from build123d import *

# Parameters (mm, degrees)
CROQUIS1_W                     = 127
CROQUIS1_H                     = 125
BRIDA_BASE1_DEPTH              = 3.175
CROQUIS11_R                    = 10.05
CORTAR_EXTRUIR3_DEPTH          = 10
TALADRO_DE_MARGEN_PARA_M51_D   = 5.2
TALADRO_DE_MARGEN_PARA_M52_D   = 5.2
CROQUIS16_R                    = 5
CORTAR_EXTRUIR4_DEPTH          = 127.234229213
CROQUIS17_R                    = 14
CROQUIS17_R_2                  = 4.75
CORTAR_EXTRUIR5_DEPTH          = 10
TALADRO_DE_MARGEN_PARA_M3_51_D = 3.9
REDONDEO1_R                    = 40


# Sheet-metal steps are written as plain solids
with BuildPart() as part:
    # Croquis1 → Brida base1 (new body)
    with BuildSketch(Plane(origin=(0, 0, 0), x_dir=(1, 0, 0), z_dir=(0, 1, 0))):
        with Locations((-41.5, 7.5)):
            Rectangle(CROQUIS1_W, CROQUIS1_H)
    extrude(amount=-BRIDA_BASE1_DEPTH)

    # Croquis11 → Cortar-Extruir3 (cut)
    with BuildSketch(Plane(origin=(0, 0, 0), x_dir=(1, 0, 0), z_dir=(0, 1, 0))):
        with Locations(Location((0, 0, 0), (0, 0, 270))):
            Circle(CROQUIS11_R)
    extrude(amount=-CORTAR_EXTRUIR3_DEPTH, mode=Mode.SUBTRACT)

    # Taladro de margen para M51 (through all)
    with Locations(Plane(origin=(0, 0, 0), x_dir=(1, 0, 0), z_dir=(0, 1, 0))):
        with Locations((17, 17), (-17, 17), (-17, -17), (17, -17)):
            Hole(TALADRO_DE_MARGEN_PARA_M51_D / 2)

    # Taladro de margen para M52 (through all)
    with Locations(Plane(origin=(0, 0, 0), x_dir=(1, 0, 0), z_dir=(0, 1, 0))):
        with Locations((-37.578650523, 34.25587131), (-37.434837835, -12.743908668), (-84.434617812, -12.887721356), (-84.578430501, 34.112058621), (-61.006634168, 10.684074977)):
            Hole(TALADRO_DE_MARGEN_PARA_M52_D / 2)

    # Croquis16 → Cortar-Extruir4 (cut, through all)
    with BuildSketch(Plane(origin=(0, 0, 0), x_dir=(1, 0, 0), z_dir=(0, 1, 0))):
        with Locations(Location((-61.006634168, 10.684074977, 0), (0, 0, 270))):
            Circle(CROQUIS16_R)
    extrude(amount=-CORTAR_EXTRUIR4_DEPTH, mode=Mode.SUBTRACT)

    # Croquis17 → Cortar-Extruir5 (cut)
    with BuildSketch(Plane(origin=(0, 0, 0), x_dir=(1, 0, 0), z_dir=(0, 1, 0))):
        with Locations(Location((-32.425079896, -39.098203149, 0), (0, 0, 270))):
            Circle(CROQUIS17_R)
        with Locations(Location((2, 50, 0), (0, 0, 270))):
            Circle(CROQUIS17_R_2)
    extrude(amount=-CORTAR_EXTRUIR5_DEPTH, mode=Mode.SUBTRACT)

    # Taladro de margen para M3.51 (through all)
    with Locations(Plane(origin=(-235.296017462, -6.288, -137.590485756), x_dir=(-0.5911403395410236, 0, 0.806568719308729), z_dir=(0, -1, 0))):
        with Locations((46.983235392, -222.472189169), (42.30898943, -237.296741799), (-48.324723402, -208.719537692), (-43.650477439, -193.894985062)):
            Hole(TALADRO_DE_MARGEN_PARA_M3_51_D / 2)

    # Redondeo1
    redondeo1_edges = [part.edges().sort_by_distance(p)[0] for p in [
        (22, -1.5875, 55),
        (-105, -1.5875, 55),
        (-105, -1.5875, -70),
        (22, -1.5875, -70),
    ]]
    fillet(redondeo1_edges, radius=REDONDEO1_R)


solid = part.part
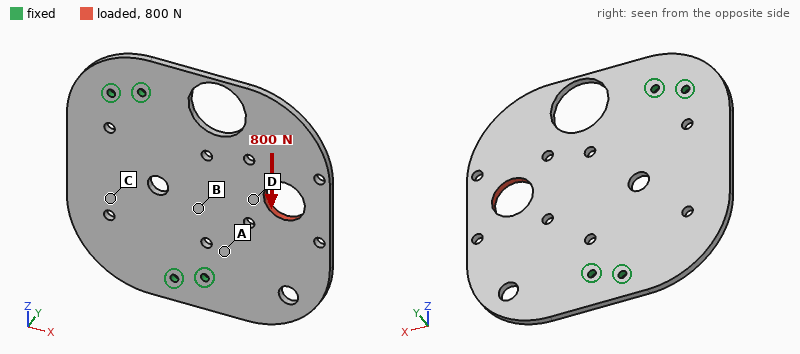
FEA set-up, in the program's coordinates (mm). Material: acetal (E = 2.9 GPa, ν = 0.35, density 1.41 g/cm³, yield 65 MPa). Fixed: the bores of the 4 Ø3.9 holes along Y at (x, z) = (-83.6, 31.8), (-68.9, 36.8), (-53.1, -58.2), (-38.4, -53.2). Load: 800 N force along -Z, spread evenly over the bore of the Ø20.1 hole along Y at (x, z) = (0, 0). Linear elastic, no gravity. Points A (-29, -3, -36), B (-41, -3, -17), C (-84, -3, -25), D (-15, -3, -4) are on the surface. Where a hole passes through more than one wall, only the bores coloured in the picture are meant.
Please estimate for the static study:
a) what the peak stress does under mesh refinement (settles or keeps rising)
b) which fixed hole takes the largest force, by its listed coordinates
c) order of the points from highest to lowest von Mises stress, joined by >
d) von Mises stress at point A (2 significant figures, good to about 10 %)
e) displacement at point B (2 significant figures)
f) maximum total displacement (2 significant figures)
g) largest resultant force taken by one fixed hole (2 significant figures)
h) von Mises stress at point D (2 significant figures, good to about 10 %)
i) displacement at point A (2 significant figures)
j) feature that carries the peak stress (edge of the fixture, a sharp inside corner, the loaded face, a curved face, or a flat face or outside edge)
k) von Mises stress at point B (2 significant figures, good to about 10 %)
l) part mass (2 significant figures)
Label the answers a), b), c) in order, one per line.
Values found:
a) keeps rising
b) (-38.4, -53.2)
c) D > A > B > C
d) 6.0 MPa
e) 0.052 mm
f) 0.30 mm
g) 540 N
h) 8.9 MPa
i) 0.067 mm
j) edge of the fixture
k) 3.7 MPa
l) 59 g
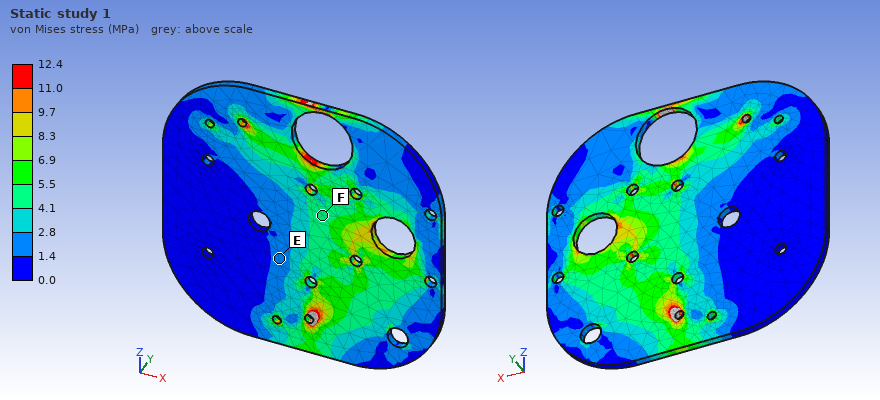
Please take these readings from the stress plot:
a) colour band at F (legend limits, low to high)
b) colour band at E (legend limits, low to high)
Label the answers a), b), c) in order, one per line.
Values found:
a) 4.1 to 5.5 MPa
b) 1.4 to 2.8 MPa
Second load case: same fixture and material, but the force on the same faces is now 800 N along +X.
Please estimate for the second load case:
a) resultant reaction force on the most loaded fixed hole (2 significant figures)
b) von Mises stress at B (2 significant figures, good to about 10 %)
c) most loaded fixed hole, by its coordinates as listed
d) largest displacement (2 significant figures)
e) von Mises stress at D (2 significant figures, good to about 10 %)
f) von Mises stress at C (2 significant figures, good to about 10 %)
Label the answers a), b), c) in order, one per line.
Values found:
a) 280 N
b) 1.8 MPa
c) (-68.9, 36.8)
d) 0.20 mm
e) 4.7 MPa
f) 1.4 MPa
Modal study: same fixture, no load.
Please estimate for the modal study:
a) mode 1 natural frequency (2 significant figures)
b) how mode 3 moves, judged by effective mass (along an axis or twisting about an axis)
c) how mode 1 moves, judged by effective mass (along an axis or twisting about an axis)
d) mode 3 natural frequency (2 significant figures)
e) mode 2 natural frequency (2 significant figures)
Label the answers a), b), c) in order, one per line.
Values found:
a) 120 Hz
b) along Y
c) along Y
d) 340 Hz
e) 290 Hz
